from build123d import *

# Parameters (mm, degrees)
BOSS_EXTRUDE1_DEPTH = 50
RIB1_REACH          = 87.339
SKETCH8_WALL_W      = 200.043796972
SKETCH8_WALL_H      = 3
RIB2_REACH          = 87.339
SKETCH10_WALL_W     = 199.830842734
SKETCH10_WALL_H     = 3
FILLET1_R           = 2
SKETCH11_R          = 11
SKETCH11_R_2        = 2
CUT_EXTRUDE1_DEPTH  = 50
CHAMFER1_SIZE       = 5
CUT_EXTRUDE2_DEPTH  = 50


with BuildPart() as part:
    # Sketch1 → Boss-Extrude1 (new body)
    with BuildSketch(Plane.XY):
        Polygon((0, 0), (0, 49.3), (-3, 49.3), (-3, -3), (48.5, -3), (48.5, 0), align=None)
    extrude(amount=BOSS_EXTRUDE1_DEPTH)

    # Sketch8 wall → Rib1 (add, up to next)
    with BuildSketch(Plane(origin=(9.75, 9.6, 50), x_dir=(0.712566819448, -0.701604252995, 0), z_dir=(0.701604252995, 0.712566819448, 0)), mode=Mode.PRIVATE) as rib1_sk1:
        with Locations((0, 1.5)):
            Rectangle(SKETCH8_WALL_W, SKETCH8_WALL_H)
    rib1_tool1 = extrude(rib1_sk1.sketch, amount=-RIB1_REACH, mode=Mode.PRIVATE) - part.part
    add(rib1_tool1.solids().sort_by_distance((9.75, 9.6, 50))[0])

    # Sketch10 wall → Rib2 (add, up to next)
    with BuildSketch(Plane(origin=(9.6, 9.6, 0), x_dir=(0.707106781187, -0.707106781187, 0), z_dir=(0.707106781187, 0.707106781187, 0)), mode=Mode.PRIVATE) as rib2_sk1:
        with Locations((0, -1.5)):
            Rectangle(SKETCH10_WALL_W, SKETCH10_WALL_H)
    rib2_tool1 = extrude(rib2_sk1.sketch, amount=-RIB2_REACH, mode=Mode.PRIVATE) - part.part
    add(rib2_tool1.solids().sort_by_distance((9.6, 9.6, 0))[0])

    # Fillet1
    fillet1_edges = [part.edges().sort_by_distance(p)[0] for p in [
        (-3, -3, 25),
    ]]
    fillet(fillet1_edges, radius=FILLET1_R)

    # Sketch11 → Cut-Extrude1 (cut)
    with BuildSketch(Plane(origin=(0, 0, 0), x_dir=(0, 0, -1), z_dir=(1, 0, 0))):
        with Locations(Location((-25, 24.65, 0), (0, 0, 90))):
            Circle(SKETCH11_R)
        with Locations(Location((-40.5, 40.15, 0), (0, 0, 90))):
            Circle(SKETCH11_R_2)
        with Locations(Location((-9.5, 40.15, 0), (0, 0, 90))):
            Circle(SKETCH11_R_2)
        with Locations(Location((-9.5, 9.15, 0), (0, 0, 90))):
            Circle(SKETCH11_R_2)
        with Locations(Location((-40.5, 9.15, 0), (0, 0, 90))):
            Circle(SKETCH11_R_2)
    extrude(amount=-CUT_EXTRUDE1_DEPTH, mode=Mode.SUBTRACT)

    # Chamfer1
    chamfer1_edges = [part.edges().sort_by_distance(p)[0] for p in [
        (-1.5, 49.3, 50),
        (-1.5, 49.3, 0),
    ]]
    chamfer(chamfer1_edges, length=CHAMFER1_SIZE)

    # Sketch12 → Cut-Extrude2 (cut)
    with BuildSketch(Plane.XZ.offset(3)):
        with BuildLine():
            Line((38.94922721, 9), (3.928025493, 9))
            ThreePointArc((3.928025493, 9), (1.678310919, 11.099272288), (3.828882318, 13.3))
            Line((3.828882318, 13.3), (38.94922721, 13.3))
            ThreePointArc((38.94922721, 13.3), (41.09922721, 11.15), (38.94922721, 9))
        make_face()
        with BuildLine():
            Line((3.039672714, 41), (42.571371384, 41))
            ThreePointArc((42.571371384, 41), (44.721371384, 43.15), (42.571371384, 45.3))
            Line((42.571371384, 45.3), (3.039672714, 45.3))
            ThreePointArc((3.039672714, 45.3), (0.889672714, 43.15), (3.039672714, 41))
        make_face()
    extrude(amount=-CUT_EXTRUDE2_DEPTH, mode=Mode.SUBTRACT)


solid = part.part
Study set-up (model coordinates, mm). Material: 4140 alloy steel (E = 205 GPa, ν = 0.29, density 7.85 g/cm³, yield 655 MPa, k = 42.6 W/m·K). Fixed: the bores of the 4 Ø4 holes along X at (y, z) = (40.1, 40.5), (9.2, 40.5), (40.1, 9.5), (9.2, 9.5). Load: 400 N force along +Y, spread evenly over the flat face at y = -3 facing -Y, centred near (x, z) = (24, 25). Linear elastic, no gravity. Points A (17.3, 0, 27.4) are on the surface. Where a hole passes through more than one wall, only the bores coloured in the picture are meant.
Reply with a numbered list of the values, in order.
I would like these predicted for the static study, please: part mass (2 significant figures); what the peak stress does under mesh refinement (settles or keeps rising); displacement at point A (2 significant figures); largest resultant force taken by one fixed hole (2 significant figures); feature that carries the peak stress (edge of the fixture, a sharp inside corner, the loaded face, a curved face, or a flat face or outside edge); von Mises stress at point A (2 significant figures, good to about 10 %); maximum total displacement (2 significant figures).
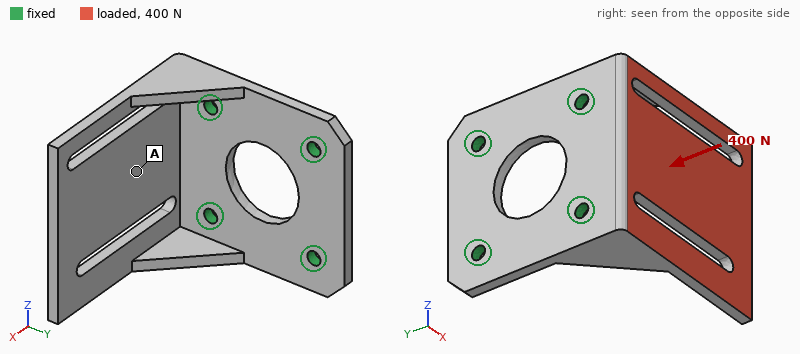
1. 110 g
2. keeps rising
3. 0.067 mm
4. 190 N
5. edge of the fixture
6. 23 MPa
7. 0.23 mm
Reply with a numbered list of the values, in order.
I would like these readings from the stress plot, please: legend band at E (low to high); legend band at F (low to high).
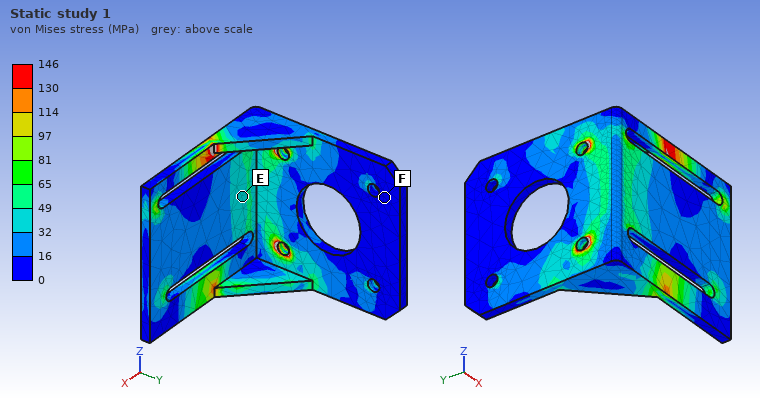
1. 32 to 49 MPa
2. 0 to 16 MPa
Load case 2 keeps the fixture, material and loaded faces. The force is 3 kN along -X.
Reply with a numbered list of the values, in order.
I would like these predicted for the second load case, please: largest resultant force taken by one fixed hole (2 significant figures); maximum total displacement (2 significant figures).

1. 1.8 kN
2. 0.33 mm
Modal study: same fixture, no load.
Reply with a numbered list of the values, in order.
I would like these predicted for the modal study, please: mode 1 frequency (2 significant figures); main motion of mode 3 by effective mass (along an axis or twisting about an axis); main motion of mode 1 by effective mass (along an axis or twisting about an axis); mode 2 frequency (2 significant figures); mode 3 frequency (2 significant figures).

1. 1200 Hz
2. along Z
3. along Y
4. 2600 Hz
5. 3800 Hz
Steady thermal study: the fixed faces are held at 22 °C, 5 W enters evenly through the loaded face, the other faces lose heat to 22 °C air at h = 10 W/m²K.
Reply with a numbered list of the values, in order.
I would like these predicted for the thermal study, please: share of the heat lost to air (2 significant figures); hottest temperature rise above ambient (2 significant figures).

1. 14 %
2. 25 K
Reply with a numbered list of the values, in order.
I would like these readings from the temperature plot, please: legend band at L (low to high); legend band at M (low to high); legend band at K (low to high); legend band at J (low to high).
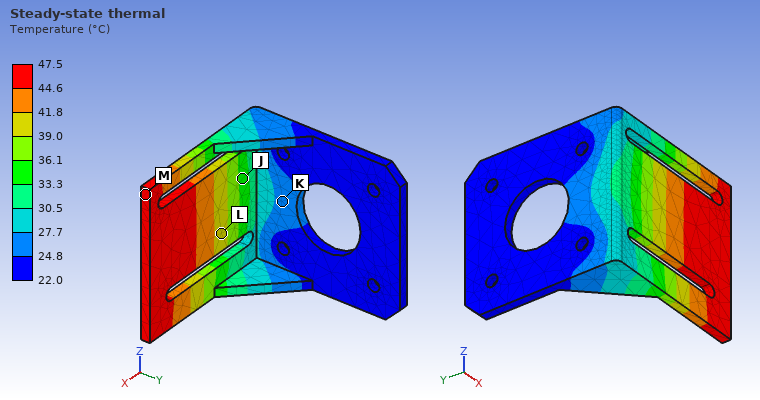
1. 39.0 to 41.8 °C
2. 44.6 to 47.5 °C
3. 24.8 to 27.7 °C
4. 33.3 to 36.1 °C
